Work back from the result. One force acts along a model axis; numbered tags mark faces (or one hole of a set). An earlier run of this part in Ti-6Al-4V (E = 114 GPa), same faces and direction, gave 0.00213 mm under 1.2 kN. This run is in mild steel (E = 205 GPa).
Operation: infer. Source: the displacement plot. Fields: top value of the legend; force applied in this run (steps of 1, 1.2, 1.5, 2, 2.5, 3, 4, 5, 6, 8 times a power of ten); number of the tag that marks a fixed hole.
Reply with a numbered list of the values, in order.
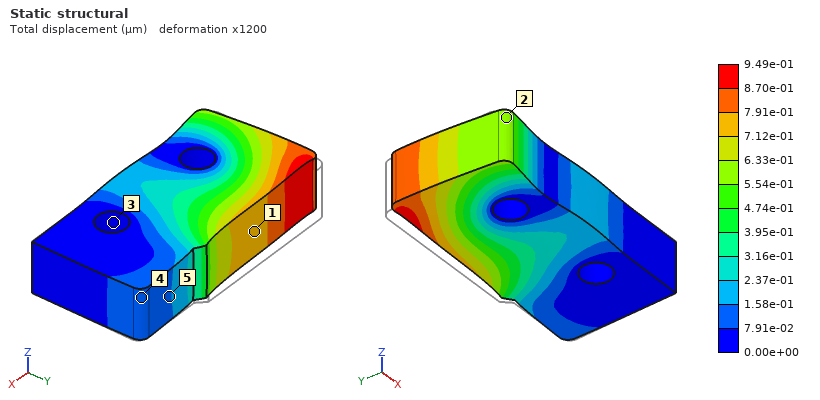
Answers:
1. 9.49e-01 µm
2. 1 kN
3. 3
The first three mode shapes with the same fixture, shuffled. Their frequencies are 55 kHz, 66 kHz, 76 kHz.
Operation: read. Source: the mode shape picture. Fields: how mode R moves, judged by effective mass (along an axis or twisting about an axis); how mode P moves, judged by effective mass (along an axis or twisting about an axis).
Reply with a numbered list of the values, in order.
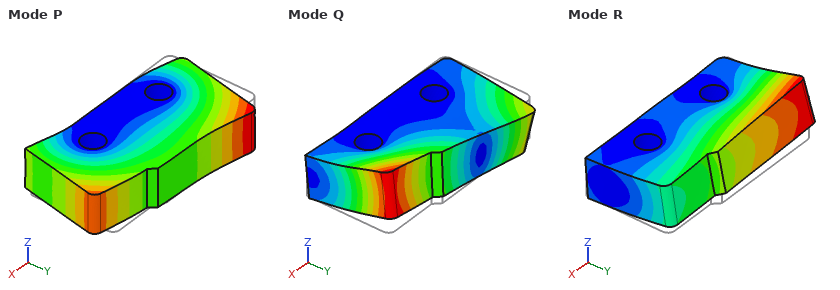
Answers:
1. along Z
2. along X
